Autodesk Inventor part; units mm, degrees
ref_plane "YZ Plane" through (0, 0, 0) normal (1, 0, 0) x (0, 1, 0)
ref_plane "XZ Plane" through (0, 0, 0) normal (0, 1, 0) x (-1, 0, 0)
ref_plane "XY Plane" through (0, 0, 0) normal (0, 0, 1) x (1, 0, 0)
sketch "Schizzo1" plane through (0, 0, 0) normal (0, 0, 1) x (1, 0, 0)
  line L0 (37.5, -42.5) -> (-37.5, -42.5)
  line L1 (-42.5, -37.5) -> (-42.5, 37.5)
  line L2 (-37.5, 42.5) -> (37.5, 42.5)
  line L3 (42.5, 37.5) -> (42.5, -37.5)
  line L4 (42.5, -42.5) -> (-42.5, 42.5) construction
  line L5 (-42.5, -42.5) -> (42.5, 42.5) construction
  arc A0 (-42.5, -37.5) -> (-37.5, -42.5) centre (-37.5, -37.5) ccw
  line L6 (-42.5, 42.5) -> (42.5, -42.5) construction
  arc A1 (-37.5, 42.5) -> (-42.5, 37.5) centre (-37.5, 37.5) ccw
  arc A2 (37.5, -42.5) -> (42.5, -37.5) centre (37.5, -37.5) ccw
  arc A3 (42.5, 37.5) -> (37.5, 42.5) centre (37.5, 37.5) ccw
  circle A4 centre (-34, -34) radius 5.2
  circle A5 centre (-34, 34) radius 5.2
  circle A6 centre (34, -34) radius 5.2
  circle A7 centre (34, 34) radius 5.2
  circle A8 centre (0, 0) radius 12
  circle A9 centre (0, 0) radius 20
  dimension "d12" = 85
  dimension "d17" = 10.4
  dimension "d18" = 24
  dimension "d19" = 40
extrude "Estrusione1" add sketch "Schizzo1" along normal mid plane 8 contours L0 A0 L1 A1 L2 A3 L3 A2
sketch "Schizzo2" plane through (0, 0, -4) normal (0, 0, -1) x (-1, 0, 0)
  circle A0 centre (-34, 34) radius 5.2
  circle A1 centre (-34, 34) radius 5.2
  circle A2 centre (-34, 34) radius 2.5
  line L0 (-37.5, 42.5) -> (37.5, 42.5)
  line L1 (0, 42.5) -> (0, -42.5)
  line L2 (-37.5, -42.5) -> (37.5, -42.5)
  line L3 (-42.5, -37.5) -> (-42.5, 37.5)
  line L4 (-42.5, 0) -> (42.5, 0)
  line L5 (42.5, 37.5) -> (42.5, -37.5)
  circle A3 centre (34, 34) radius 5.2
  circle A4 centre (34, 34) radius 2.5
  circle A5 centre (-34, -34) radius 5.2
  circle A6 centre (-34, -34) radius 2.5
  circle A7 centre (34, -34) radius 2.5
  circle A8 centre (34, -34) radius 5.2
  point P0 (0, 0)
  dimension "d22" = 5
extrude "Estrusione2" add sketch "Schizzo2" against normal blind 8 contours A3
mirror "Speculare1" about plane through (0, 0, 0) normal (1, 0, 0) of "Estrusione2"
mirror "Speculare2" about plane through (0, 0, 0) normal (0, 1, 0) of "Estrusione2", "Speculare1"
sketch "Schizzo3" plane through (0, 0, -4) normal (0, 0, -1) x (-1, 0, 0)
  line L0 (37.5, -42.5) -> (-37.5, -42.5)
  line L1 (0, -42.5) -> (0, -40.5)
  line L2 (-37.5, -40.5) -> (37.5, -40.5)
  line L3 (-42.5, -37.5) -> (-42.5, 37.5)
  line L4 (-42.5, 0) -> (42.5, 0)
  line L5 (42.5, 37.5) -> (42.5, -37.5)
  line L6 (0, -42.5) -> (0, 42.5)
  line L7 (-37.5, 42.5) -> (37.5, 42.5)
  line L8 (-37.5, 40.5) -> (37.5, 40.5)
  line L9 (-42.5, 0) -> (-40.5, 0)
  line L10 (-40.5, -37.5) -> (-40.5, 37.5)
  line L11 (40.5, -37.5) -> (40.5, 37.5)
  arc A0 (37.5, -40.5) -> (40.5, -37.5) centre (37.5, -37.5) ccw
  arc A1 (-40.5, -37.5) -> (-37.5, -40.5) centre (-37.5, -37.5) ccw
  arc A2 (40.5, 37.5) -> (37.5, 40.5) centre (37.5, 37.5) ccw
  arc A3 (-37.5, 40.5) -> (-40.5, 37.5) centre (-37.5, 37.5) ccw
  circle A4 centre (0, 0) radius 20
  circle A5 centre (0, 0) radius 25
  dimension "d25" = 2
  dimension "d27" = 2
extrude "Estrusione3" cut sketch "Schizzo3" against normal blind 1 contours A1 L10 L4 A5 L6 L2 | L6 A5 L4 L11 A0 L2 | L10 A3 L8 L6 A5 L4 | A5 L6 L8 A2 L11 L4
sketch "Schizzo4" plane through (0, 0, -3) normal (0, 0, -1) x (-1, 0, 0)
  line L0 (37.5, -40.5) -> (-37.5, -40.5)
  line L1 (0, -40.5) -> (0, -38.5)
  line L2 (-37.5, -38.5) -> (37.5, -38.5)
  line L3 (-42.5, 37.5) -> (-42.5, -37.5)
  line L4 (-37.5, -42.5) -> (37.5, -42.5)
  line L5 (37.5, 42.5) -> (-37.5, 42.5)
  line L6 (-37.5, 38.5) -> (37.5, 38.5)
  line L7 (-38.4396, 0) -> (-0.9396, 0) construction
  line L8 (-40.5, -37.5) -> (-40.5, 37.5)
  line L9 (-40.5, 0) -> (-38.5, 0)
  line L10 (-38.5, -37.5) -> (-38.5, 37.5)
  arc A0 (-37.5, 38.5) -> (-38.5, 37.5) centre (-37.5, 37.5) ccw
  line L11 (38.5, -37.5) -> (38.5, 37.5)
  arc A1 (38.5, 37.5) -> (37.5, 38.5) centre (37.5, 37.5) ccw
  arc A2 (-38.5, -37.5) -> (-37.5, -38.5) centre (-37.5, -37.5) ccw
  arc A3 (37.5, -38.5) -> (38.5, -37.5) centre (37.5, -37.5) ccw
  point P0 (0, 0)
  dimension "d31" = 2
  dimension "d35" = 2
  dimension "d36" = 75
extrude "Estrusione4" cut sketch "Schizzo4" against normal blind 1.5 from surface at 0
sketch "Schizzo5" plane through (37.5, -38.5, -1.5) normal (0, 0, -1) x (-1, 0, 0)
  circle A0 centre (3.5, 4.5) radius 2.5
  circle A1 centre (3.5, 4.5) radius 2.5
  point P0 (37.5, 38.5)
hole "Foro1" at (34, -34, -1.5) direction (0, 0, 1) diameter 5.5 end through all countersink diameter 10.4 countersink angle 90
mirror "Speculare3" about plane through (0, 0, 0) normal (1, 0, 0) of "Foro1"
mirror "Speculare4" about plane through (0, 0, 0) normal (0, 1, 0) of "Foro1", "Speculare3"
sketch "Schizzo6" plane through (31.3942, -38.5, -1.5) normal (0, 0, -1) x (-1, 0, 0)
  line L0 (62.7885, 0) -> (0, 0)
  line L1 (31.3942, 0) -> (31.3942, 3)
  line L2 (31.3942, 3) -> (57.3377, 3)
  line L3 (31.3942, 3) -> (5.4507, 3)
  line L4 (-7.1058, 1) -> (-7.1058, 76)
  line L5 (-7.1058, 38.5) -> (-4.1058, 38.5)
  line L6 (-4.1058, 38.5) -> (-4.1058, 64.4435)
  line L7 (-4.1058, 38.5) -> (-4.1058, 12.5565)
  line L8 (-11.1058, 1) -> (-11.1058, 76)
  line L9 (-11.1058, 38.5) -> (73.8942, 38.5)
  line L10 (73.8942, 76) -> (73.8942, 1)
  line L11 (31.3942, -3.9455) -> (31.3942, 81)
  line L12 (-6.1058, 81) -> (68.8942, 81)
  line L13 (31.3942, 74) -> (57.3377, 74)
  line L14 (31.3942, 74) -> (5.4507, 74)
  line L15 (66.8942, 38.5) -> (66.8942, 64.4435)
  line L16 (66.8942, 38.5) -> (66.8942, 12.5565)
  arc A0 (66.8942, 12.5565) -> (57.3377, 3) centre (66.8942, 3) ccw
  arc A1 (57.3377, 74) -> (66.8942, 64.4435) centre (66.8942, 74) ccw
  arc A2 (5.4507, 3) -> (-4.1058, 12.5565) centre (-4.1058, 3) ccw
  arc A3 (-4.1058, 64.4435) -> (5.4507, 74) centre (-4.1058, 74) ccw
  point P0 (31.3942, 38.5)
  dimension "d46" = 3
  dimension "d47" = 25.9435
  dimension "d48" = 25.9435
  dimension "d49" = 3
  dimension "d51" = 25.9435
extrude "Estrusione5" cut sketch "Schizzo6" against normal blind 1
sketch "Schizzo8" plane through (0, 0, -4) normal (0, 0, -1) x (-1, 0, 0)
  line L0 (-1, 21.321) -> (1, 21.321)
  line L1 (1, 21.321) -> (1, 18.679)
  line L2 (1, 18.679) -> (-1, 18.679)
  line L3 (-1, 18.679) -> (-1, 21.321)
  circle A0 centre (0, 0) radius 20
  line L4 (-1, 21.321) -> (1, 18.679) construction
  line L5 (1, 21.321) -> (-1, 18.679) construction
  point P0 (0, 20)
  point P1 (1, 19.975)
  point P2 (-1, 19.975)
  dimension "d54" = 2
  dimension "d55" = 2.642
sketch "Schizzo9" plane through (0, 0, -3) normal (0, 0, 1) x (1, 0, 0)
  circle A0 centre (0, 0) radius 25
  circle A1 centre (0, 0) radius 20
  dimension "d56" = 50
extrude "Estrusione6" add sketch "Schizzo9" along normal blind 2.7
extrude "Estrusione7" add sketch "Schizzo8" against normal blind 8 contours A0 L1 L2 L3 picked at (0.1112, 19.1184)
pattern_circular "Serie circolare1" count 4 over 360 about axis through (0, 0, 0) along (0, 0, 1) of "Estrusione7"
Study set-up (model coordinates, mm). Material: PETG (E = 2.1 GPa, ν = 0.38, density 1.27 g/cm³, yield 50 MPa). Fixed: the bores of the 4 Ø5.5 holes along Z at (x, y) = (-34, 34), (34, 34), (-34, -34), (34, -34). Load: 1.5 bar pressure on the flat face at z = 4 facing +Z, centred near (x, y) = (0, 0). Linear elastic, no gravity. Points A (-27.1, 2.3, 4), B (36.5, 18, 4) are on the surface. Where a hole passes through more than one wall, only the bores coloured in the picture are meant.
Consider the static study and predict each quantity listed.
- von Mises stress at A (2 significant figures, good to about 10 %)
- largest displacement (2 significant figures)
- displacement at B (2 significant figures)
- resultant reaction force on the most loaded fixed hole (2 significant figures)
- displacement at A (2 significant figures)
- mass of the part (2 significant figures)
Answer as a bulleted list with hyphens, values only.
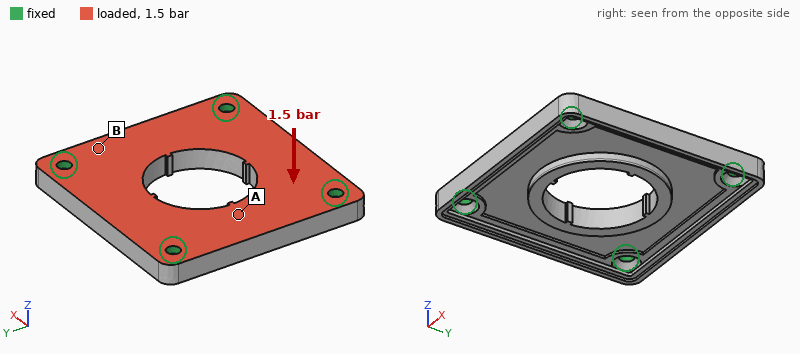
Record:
- 4.7 MPa
- 0.55 mm
- 0.21 mm
- 250 N
- 0.46 mm
- 43 g
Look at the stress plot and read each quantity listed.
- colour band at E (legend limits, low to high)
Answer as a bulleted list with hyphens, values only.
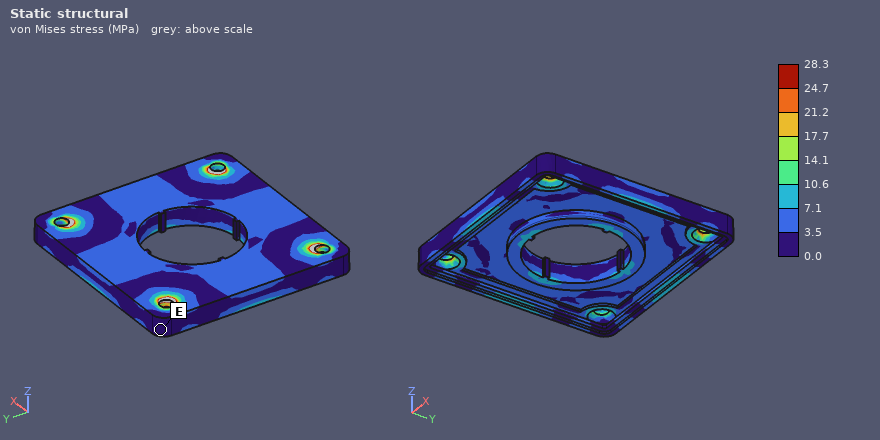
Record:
- 0.0 to 3.5 MPa
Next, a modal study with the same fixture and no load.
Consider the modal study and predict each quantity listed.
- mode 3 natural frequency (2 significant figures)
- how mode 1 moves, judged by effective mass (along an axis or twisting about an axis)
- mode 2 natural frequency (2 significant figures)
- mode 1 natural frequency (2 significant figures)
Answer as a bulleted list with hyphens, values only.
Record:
- 1500 Hz
- along Z
- 1500 Hz
- 1200 Hz
